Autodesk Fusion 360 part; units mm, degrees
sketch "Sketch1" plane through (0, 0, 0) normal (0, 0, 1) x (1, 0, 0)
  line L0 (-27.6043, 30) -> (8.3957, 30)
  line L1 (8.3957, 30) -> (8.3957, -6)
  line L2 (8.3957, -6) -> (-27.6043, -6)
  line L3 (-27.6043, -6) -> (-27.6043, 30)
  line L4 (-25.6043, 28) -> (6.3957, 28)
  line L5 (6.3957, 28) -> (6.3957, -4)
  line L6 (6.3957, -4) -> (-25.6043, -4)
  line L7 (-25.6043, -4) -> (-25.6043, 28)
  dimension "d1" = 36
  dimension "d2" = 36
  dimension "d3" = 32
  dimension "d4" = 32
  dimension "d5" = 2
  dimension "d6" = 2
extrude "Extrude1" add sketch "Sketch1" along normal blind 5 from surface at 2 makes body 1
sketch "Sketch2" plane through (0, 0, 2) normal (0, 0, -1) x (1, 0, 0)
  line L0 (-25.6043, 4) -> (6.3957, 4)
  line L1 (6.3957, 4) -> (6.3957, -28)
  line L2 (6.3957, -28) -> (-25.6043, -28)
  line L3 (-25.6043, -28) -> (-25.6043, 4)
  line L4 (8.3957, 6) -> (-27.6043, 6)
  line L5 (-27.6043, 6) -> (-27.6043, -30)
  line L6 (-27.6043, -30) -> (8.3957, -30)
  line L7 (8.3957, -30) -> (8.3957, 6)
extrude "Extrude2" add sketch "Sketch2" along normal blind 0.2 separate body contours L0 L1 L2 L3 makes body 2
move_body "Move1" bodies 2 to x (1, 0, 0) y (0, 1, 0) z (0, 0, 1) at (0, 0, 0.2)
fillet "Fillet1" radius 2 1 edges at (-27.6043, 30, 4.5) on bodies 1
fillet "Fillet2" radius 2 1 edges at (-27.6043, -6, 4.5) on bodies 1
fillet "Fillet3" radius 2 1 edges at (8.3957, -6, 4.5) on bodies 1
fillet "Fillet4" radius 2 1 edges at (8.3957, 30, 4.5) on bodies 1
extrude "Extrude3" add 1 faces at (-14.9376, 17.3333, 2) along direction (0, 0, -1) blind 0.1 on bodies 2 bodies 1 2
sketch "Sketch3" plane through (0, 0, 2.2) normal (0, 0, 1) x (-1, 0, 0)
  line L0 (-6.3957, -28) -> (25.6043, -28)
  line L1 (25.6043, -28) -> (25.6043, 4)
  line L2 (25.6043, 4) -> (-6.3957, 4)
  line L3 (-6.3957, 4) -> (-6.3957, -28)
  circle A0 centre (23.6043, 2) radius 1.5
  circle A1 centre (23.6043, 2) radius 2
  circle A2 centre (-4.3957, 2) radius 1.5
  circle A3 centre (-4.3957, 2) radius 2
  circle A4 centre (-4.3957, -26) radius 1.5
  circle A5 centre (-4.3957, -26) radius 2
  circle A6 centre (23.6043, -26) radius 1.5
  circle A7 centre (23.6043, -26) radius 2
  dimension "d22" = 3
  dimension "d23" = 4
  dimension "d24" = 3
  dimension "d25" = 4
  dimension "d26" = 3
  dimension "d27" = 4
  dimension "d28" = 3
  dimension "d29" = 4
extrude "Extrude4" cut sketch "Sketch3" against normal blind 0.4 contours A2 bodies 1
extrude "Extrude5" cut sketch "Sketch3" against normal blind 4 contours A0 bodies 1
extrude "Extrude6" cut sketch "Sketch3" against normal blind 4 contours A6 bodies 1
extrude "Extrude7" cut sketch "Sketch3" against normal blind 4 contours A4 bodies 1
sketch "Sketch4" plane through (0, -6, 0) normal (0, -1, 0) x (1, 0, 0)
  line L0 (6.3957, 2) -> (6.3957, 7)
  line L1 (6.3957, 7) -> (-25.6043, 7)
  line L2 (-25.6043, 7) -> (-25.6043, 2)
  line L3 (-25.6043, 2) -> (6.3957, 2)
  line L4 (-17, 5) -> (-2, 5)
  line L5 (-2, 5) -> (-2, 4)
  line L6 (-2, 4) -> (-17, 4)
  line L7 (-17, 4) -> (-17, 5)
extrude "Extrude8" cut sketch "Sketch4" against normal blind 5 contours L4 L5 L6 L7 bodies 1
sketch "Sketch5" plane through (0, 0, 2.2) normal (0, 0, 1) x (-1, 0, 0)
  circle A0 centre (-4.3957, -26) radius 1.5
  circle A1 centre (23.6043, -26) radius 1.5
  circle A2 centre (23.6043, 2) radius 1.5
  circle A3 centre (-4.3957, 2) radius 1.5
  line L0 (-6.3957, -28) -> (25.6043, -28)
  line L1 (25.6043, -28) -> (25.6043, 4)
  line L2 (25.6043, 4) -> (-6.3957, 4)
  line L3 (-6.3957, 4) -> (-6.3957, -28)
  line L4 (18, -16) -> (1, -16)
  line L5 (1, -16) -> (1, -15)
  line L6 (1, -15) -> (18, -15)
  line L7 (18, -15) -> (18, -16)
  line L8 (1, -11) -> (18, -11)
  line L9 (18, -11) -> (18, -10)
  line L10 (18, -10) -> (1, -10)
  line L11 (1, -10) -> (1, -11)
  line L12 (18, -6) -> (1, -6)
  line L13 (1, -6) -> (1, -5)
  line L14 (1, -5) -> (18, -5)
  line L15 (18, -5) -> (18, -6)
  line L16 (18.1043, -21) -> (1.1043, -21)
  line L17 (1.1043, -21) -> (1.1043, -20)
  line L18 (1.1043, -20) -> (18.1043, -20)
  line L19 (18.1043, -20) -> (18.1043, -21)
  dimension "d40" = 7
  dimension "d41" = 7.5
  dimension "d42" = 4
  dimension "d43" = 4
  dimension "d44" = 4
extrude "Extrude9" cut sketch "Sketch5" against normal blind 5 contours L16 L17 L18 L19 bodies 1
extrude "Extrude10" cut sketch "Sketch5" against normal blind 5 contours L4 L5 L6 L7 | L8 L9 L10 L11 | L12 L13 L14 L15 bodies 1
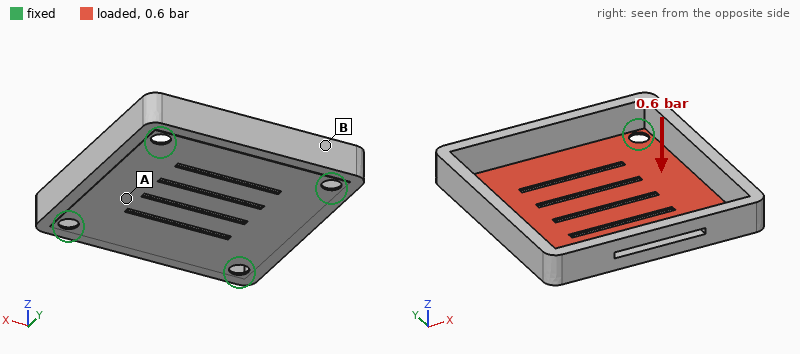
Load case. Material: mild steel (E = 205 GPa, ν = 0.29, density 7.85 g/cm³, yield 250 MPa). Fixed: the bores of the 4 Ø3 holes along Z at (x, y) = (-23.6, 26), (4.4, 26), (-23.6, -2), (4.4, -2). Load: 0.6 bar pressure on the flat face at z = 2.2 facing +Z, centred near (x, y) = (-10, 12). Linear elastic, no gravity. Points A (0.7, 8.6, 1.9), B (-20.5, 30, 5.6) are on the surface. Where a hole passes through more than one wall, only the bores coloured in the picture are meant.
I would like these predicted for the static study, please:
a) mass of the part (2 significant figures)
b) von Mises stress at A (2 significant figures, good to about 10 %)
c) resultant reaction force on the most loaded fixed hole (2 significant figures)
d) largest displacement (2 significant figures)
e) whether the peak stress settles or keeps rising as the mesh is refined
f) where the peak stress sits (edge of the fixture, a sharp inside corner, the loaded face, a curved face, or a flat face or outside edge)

12 g
70 MPa
21 N
0.25 mm
keeps rising
a sharp inside corner
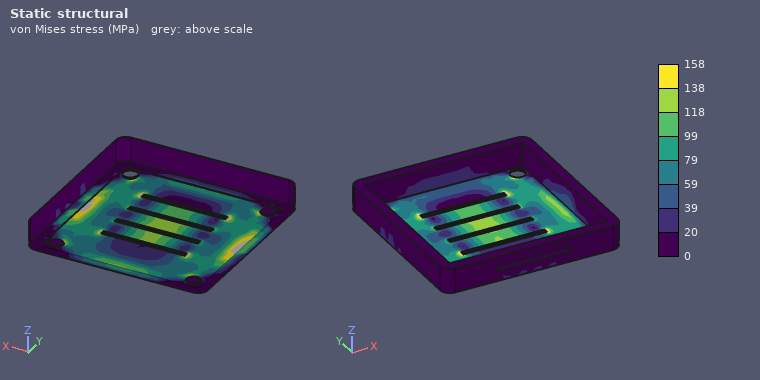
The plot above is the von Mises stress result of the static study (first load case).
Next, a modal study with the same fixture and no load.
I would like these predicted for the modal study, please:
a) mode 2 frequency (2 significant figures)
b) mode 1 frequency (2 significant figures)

3000 Hz
2100 Hz
